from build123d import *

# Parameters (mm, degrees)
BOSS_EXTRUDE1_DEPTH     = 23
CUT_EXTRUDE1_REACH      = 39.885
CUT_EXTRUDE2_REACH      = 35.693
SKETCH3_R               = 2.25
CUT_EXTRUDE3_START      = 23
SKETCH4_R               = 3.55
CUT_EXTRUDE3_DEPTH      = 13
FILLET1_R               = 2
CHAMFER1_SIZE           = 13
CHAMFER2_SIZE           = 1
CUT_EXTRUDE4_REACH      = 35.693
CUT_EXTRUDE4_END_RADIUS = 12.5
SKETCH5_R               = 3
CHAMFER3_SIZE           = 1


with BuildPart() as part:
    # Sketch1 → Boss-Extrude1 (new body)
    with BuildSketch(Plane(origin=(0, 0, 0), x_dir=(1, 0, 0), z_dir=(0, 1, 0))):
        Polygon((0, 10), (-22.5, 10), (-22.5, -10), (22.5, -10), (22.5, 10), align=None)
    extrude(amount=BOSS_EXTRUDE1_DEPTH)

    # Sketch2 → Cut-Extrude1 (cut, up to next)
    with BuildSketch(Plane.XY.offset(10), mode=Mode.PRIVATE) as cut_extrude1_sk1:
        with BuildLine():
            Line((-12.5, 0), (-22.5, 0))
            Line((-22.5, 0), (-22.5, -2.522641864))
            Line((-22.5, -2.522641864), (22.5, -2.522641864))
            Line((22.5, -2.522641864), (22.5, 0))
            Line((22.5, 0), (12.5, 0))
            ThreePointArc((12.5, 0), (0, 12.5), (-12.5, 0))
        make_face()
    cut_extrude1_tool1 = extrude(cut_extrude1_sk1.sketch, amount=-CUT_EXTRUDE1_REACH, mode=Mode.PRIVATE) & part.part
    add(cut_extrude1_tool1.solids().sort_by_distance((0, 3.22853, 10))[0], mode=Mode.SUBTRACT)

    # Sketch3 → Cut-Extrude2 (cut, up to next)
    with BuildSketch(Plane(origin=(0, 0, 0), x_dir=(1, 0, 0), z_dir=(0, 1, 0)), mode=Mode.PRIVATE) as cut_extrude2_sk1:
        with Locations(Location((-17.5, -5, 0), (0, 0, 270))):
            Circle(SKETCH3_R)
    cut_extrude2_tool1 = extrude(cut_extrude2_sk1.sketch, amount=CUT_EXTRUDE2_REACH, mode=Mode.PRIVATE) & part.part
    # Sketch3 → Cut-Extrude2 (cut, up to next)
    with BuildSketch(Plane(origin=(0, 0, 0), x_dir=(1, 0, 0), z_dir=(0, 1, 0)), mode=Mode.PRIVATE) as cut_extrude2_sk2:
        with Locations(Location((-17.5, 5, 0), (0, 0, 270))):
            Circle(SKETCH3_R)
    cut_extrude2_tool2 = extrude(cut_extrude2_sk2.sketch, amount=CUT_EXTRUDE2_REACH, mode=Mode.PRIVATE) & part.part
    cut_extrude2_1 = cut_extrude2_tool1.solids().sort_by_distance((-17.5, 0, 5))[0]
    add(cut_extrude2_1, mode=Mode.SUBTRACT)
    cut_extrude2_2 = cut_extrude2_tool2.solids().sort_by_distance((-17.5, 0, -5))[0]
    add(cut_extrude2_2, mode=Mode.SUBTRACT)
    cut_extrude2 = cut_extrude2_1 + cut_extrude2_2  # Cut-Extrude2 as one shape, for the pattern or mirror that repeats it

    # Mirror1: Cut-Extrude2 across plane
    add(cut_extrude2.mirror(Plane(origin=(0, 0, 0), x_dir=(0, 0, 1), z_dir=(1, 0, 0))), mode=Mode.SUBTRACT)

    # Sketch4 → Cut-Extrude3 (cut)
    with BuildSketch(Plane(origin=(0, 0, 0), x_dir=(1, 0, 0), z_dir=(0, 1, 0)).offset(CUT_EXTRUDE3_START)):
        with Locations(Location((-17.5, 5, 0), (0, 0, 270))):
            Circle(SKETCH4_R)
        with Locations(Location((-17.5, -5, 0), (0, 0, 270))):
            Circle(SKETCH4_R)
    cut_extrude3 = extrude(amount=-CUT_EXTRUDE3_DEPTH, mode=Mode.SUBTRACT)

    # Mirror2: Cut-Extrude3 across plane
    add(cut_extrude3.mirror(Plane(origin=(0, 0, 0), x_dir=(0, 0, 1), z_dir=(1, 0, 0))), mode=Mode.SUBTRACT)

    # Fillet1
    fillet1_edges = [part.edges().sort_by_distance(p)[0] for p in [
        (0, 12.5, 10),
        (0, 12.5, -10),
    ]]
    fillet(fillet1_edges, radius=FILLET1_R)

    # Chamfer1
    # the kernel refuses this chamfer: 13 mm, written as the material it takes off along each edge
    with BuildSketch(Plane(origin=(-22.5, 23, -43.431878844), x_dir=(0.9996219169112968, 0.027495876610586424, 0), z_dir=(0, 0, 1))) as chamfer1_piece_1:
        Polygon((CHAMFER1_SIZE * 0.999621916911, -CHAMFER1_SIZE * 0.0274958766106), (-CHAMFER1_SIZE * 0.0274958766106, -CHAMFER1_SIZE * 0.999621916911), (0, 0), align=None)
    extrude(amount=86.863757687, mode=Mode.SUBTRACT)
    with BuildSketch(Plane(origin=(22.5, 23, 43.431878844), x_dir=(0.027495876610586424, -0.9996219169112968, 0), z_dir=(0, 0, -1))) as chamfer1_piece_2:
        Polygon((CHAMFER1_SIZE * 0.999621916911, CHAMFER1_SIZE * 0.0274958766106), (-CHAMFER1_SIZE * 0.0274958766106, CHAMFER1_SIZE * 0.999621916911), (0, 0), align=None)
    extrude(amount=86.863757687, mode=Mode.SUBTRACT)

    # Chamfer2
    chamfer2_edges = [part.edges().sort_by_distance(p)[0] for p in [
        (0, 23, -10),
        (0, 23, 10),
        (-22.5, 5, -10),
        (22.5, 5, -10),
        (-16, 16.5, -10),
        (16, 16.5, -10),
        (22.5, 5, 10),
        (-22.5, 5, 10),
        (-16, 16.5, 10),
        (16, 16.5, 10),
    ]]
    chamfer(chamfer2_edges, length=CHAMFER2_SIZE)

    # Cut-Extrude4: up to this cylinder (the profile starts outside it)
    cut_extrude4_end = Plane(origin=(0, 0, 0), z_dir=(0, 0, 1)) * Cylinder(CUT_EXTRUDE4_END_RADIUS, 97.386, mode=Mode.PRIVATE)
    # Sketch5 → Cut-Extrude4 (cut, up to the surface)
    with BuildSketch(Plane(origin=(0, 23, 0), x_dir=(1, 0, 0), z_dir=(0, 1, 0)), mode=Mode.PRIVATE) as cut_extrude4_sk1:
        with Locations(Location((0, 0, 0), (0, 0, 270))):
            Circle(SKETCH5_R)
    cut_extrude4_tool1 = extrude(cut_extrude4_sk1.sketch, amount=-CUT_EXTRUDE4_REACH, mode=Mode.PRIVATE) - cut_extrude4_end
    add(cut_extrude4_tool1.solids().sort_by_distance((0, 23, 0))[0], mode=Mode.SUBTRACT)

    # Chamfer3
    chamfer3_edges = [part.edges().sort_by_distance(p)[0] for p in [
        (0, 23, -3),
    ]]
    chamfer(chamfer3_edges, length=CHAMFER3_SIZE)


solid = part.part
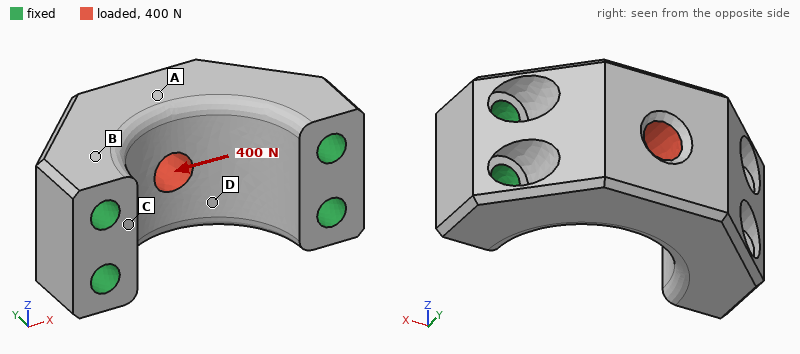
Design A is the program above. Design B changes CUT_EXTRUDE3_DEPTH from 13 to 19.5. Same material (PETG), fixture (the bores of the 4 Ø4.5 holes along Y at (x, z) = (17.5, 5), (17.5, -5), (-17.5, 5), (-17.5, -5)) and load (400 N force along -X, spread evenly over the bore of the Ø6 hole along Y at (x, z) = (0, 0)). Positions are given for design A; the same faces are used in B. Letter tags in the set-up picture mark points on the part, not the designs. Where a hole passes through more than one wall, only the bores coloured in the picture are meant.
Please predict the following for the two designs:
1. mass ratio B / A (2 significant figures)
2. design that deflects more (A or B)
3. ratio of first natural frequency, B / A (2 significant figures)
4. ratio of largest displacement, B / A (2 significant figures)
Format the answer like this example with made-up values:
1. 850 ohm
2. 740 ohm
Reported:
1. 0.94
2. B
3. 0.58
4. 2.5
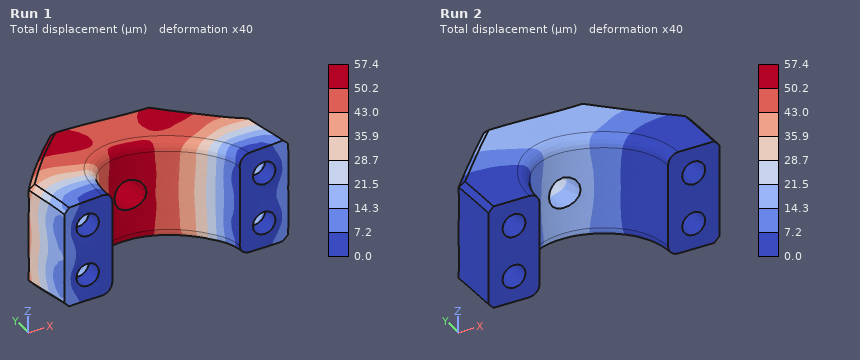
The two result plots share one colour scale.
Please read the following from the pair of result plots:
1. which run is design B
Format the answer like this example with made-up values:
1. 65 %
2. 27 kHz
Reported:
1. Run 1
